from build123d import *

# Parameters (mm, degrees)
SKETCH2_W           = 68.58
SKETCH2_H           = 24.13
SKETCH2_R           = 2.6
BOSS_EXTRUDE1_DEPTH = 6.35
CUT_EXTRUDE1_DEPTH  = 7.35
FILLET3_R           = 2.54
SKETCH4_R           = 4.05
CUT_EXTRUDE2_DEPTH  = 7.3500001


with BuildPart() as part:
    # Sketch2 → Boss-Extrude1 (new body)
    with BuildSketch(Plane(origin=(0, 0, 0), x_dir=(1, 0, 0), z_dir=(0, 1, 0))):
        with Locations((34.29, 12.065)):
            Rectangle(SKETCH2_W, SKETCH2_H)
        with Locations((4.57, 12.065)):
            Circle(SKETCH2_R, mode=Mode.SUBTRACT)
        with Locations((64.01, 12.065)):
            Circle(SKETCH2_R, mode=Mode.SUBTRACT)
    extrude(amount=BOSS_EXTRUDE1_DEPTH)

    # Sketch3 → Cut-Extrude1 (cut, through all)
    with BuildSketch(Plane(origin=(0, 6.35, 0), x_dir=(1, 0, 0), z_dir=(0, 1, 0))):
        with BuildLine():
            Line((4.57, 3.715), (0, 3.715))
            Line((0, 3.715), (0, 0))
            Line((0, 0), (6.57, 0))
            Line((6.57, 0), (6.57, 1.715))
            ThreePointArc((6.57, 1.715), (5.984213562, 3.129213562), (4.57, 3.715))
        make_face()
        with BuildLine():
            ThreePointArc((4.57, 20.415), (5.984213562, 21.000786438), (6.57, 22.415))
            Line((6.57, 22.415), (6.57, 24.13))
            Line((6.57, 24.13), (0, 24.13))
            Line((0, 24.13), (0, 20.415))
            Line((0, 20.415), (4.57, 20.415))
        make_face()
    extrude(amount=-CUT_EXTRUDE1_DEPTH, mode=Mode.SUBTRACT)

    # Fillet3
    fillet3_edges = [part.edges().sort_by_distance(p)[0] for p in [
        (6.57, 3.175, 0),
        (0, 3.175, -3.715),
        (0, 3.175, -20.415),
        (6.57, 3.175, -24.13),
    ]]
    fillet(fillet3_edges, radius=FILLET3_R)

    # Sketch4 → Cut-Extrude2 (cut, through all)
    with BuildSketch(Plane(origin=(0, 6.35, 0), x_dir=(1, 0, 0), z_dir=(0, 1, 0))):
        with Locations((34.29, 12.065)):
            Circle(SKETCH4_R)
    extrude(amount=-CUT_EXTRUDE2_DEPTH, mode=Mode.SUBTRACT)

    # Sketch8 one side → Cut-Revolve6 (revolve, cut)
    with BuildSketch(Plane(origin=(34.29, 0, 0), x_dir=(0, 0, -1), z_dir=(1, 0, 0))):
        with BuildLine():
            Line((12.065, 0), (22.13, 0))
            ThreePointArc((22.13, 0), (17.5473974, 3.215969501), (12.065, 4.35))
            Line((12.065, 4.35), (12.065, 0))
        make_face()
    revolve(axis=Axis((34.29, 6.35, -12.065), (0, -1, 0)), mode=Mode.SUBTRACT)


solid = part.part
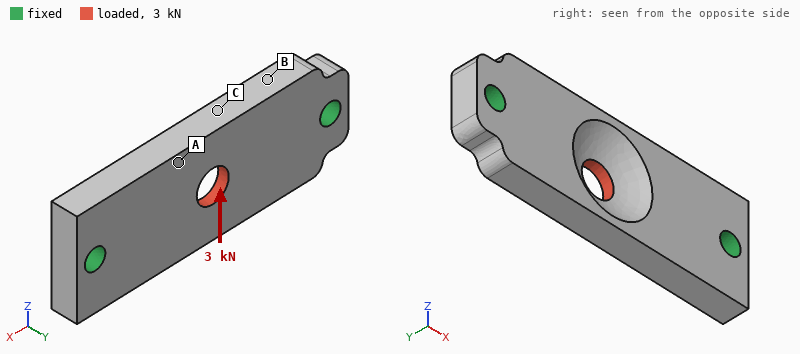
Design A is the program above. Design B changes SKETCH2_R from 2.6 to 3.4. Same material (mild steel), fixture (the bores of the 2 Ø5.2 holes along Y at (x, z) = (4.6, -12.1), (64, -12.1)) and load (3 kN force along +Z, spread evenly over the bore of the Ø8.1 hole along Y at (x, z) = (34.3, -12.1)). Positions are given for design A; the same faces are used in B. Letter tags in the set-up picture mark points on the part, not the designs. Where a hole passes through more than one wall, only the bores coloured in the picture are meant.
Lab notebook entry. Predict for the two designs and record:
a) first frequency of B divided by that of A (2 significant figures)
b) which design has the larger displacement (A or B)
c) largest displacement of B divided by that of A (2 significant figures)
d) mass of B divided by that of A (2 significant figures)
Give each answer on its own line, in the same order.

1.1
A
0.89
0.98
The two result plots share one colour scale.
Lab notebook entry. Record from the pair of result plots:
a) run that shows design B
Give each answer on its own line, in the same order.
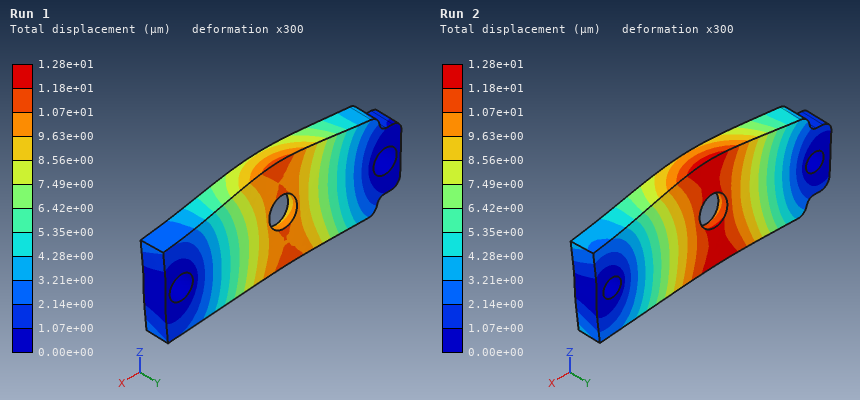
Run 1
